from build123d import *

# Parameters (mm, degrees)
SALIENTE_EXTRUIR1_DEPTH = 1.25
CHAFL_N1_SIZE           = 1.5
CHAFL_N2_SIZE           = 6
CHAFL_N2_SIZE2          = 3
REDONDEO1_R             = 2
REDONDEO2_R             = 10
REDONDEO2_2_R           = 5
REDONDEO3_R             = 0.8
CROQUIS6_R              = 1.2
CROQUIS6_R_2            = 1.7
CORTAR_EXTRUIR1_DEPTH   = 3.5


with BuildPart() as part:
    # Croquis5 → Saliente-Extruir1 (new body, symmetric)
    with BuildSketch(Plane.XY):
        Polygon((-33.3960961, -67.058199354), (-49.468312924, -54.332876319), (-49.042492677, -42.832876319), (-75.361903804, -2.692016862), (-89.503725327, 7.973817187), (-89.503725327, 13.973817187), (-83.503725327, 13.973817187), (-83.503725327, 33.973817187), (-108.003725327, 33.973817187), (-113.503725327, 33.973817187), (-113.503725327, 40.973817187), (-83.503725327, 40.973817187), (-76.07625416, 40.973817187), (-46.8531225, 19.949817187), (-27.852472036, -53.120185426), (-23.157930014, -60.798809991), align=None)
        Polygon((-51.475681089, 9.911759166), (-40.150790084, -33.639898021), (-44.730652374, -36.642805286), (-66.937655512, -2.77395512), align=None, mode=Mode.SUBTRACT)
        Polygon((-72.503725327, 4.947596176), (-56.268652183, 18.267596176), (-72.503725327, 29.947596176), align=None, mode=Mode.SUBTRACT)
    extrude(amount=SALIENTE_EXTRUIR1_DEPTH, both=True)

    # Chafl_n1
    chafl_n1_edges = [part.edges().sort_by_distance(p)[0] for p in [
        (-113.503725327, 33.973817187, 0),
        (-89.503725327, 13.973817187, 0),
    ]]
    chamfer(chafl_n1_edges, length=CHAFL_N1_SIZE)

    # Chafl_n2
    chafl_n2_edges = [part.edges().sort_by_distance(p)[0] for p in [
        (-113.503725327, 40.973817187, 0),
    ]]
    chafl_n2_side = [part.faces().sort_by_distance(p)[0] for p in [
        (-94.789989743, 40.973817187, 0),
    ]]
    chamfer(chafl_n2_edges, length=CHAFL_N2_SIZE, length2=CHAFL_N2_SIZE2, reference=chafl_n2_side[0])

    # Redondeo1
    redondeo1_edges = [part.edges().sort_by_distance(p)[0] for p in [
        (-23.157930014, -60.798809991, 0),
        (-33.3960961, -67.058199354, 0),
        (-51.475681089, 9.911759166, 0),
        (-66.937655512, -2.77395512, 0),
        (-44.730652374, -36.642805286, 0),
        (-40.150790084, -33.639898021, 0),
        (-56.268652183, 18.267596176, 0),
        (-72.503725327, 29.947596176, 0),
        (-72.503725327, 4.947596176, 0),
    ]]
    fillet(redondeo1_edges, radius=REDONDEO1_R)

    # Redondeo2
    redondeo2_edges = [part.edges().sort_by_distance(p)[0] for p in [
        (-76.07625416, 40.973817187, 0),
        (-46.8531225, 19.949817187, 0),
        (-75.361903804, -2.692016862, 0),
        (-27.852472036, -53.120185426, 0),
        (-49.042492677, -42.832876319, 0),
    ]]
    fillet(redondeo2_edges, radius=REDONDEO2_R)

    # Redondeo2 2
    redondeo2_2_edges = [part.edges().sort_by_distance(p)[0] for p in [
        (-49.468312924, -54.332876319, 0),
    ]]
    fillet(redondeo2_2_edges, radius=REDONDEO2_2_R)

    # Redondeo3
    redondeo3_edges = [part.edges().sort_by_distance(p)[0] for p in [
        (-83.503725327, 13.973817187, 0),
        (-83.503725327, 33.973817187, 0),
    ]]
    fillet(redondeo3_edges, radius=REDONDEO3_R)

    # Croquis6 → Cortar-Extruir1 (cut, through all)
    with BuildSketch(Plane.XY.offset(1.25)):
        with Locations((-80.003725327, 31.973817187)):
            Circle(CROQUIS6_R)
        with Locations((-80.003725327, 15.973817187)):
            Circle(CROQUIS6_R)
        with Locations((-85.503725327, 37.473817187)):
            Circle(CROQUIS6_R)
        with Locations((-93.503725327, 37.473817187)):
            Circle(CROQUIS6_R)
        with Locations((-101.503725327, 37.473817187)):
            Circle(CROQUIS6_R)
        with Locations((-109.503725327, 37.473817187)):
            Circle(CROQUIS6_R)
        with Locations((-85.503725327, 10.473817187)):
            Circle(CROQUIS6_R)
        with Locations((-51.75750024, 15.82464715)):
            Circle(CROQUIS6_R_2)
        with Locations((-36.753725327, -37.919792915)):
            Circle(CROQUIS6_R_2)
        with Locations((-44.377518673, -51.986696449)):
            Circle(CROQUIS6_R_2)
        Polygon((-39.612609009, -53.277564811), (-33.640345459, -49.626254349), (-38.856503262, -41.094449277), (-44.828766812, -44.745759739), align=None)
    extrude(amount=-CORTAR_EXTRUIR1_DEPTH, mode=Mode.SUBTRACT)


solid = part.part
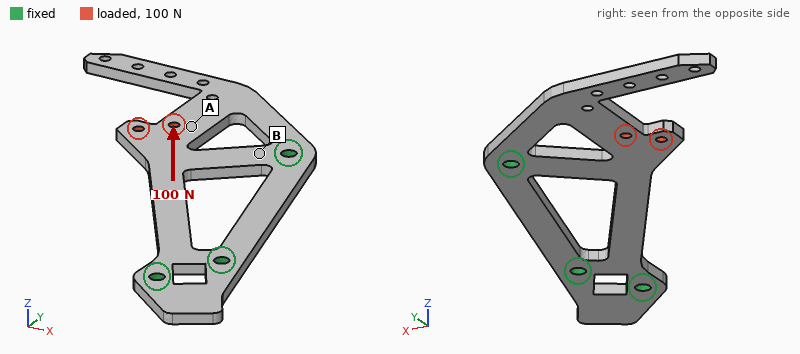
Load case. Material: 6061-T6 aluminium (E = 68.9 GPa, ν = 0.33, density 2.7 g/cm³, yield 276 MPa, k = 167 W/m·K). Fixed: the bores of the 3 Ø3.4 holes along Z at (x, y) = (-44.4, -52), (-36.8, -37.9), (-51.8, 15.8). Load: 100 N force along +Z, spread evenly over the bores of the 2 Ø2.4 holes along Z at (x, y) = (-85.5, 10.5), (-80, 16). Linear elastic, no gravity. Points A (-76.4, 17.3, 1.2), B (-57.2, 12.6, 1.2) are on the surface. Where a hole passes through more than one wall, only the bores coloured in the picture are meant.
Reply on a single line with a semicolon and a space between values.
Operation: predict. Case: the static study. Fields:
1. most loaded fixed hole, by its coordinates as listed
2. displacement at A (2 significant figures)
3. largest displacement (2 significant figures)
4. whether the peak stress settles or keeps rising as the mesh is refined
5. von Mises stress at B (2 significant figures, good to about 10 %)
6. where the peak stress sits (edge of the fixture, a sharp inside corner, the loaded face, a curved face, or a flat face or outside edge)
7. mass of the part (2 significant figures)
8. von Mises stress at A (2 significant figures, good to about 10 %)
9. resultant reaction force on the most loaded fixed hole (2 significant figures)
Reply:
(-51.8, 15.8); 0.46 mm; 1.4 mm; keeps rising; 120 MPa; edge of the fixture; 15 g; 24 MPa; 100 N
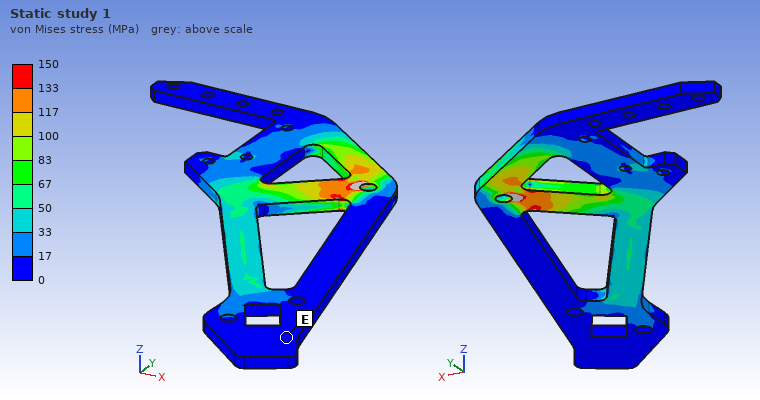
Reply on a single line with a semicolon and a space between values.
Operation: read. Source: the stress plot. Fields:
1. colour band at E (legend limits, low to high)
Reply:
0 to 17 MPa
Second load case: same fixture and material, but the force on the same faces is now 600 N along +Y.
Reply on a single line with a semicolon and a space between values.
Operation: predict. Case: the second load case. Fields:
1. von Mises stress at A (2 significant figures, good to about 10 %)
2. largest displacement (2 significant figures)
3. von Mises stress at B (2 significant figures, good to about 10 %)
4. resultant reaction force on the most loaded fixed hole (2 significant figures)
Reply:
18 MPa; 83 µm; 17 MPa; 380 N
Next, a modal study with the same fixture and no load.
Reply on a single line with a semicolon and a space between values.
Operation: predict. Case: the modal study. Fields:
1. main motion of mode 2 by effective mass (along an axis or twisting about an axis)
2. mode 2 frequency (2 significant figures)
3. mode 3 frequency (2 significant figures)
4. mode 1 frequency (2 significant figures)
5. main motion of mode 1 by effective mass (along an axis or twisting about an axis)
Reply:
along Z; 1700 Hz; 2400 Hz; 660 Hz; along Z
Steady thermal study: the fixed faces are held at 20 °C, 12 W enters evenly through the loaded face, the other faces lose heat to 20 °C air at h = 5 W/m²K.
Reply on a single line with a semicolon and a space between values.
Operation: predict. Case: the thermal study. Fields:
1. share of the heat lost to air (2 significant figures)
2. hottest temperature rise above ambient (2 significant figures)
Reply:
4.6 %; 60 K
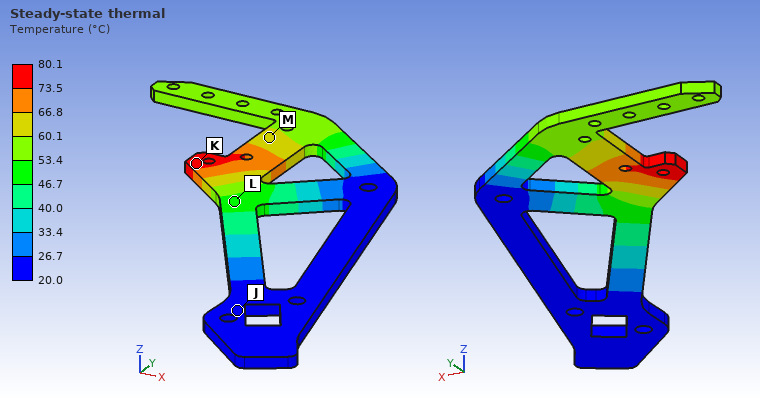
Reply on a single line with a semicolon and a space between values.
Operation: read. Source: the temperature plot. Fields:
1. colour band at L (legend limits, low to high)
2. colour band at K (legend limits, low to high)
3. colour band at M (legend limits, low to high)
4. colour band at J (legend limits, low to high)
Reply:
46.7 to 53.4 °C; 73.5 to 80.1 °C; 60.1 to 66.8 °C; 20.0 to 26.7 °C
